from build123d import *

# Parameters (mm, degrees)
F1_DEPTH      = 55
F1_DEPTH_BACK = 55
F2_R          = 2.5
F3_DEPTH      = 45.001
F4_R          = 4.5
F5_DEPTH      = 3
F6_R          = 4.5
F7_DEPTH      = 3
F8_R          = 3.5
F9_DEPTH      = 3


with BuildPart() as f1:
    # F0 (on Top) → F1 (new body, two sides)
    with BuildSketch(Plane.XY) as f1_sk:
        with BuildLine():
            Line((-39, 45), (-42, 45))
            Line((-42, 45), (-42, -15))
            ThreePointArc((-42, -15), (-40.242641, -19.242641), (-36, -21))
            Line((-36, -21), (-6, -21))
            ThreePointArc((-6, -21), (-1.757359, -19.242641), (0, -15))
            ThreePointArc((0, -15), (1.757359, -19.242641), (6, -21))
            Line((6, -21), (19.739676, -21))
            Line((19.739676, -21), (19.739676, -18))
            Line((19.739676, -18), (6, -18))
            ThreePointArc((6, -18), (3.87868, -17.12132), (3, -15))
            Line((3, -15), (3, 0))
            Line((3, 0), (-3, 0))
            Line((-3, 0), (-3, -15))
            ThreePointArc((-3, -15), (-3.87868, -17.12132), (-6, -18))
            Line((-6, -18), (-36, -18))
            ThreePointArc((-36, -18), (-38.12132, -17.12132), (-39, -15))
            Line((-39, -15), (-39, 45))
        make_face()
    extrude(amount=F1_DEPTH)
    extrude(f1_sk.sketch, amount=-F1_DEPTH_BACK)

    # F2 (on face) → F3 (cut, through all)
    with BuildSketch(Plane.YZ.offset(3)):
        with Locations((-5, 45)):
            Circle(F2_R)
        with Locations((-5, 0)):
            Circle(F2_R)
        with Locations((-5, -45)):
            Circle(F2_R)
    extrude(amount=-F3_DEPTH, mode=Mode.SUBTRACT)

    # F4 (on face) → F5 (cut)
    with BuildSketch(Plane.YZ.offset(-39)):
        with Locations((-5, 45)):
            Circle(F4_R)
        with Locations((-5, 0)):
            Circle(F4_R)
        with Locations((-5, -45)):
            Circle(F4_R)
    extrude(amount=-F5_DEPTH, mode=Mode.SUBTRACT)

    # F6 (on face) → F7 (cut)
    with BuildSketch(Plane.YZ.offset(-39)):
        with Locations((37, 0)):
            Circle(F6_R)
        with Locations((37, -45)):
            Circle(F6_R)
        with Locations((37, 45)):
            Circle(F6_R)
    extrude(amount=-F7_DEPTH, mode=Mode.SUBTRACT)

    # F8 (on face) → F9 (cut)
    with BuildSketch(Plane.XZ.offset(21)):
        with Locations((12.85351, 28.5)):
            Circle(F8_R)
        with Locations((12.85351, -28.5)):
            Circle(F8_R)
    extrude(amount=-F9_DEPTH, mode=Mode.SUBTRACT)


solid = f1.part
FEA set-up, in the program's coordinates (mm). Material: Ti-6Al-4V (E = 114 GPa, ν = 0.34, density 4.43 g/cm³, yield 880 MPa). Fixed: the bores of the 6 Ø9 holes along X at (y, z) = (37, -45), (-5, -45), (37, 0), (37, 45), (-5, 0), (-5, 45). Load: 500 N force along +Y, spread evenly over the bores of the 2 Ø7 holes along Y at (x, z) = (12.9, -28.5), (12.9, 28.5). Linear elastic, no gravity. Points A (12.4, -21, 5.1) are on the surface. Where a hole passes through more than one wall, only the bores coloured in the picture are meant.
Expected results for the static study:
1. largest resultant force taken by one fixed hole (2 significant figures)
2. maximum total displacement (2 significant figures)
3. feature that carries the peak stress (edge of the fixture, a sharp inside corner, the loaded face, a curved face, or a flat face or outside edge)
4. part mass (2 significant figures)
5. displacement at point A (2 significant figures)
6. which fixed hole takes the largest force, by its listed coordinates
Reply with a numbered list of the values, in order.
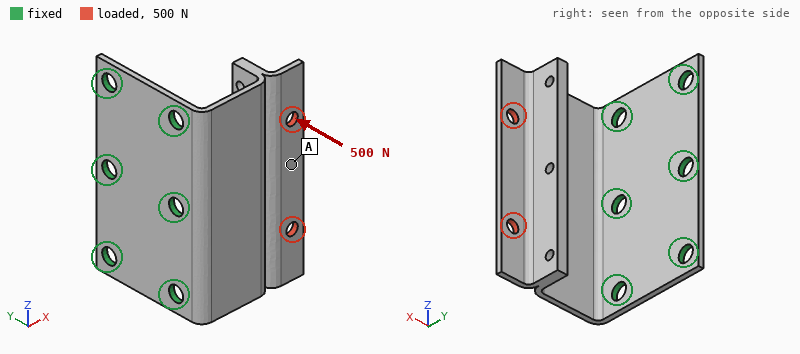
1. 210 N
2. 1.6 mm
3. a flat face or outside edge
4. 220 g
5. 1.3 mm
6. (-5, 0)
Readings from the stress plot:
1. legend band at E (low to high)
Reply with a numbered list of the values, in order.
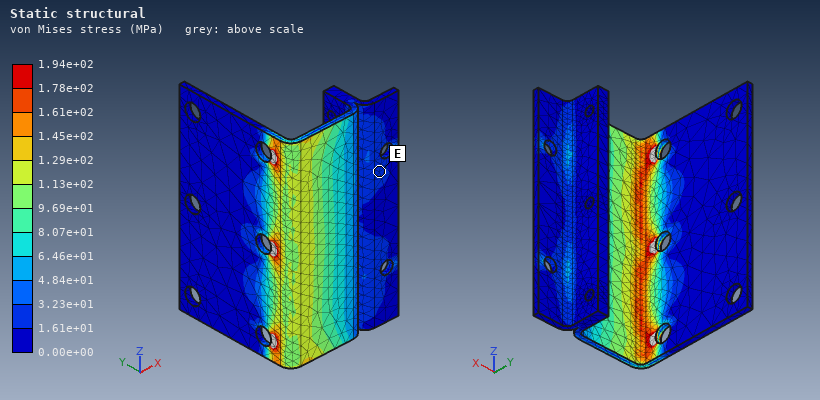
1. 1.61e+01 to 3.23e+01 MPa
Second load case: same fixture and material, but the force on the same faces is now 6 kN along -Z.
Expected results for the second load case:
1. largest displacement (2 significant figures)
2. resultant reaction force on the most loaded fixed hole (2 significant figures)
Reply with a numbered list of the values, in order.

1. 0.63 mm
2. 4.1 kN
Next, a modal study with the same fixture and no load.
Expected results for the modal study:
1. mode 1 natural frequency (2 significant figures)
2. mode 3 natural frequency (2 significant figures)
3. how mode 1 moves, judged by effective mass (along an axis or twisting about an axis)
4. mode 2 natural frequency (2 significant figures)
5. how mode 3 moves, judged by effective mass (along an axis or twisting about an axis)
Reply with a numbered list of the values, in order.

1. 410 Hz
2. 2100 Hz
3. along Y
4. 860 Hz
5. along X
